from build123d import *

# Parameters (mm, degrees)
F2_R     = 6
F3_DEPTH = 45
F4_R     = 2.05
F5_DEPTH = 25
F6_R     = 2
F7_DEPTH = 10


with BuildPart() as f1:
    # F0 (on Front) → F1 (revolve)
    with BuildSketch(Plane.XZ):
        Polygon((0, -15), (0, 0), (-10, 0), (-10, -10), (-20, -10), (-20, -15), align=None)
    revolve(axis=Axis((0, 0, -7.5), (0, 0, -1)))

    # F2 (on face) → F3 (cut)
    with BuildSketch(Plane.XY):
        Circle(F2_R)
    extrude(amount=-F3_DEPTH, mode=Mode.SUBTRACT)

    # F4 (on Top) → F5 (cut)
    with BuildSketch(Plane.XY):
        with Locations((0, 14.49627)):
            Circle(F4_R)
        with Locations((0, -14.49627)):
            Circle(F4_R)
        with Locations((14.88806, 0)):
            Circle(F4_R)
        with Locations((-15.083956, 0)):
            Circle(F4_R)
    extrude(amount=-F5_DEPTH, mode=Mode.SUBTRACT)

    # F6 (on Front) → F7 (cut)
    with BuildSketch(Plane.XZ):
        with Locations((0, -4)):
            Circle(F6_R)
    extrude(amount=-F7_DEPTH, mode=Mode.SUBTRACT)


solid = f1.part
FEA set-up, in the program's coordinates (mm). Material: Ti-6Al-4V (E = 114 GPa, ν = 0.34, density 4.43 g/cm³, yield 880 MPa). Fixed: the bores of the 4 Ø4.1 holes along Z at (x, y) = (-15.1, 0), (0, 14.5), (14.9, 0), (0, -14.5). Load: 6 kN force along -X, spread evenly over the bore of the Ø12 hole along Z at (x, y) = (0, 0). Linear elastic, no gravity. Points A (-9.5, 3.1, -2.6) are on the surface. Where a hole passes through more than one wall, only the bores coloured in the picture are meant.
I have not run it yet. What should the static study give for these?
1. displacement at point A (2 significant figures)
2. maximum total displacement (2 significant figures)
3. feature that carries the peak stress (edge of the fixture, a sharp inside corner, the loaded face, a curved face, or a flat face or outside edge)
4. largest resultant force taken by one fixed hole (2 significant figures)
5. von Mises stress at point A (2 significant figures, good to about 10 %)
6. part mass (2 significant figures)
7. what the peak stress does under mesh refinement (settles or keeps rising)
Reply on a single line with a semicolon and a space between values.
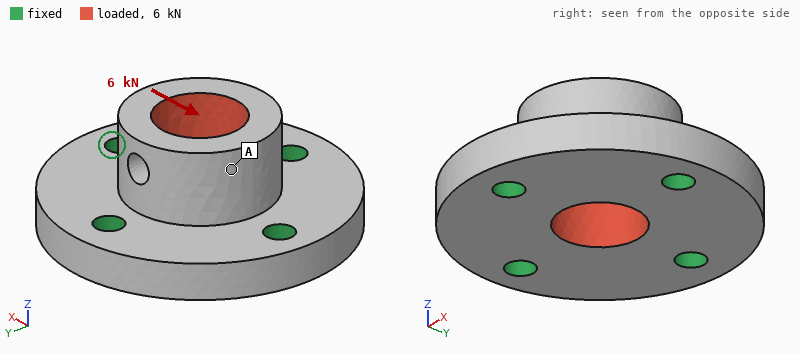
10 µm; 13 µm; edge of the fixture; 2.1 kN; 15 MPa; 33 g; keeps rising
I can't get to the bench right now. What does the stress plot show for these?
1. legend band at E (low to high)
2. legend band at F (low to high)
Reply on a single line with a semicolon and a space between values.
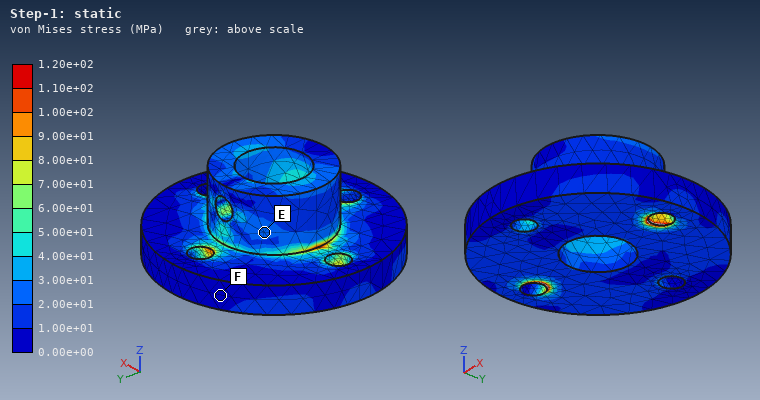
2.00e+01 to 3.00e+01 MPa; 0.00e+00 to 1.00e+01 MPa
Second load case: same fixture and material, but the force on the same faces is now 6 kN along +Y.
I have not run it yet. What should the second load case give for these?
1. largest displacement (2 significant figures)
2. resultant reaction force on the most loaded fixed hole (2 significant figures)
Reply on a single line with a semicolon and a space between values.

12 µm; 2.2 kN
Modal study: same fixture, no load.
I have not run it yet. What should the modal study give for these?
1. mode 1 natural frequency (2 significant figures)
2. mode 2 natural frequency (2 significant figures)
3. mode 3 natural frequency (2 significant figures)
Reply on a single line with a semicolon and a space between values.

33 kHz; 34 kHz; 36 kHz
